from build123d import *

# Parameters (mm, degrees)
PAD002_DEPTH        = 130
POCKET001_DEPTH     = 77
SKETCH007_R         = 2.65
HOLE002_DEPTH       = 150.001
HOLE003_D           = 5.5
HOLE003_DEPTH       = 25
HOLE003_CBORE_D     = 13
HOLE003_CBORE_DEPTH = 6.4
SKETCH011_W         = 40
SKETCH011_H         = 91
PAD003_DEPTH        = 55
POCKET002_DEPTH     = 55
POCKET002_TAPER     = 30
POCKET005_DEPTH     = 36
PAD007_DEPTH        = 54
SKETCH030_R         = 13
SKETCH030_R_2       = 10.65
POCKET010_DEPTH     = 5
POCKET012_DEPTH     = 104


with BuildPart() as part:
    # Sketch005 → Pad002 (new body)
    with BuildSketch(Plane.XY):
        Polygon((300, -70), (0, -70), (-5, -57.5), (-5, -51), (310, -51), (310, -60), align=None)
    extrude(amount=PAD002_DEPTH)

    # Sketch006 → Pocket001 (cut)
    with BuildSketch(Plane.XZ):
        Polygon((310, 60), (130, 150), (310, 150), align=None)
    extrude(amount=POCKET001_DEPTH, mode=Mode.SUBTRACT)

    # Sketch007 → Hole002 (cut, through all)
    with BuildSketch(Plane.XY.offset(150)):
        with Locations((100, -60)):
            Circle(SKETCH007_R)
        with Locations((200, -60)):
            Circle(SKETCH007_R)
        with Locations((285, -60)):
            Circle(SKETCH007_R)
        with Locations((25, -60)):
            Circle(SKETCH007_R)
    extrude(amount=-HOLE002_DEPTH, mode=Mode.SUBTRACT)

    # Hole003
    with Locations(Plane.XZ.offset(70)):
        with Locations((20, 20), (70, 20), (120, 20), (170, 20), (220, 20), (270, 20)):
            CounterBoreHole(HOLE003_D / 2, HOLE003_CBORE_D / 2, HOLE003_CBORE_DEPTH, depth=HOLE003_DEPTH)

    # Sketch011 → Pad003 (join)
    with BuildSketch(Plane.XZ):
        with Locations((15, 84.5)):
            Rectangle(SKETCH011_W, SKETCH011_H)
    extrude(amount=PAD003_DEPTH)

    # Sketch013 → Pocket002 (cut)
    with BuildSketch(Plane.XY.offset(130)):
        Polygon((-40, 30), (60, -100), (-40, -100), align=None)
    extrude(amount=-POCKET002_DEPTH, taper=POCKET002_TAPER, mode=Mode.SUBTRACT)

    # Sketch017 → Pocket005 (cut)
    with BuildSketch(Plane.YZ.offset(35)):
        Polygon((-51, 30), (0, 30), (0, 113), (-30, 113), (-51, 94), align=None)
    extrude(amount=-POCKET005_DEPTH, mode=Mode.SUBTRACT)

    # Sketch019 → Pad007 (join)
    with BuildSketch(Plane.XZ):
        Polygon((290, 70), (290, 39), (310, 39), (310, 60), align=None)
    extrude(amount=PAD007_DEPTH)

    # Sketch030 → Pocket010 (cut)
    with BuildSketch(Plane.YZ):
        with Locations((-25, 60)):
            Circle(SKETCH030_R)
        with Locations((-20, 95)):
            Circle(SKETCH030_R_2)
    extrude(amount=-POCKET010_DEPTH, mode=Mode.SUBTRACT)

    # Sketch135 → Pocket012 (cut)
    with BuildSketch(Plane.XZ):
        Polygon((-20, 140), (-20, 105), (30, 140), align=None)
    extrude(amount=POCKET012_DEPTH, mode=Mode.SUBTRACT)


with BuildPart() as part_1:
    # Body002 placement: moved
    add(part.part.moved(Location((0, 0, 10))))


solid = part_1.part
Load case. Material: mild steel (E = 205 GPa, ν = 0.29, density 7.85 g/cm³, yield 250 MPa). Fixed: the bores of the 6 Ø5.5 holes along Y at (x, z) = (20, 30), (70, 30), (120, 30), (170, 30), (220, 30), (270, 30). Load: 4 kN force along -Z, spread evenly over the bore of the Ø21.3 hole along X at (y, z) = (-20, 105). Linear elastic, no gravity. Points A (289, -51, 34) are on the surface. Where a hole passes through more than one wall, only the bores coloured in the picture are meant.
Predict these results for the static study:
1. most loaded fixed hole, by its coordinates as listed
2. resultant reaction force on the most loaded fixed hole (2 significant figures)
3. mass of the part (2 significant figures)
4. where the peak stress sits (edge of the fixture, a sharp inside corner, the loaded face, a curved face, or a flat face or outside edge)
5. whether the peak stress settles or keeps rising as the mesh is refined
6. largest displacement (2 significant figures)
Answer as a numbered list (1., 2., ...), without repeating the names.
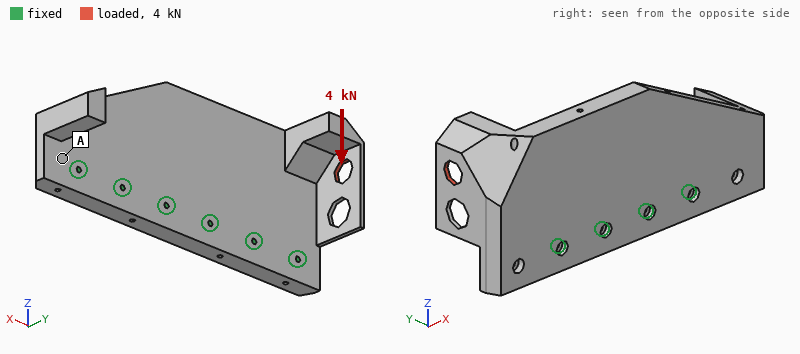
1. (20, 30)
2. 3.7 kN
3. 5.6 kg
4. edge of the fixture
5. keeps rising
6. 0.11 mm
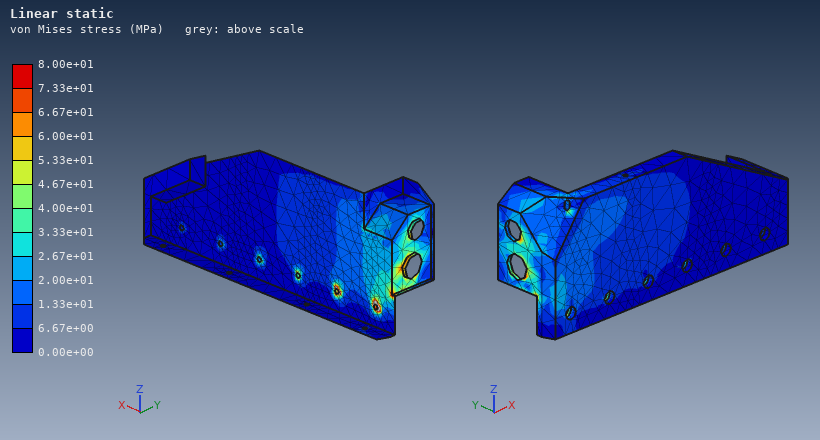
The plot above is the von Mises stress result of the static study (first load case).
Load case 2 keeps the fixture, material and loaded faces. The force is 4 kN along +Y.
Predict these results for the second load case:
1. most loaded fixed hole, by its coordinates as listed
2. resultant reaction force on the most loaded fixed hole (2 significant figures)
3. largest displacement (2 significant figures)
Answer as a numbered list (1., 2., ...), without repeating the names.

1. (20, 30)
2. 4.3 kN
3. 0.18 mm
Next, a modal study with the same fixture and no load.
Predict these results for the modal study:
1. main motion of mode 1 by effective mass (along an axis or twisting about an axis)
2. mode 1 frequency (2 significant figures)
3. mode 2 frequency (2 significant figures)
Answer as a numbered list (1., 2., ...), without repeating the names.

1. along Y
2. 860 Hz
3. 1500 Hz
